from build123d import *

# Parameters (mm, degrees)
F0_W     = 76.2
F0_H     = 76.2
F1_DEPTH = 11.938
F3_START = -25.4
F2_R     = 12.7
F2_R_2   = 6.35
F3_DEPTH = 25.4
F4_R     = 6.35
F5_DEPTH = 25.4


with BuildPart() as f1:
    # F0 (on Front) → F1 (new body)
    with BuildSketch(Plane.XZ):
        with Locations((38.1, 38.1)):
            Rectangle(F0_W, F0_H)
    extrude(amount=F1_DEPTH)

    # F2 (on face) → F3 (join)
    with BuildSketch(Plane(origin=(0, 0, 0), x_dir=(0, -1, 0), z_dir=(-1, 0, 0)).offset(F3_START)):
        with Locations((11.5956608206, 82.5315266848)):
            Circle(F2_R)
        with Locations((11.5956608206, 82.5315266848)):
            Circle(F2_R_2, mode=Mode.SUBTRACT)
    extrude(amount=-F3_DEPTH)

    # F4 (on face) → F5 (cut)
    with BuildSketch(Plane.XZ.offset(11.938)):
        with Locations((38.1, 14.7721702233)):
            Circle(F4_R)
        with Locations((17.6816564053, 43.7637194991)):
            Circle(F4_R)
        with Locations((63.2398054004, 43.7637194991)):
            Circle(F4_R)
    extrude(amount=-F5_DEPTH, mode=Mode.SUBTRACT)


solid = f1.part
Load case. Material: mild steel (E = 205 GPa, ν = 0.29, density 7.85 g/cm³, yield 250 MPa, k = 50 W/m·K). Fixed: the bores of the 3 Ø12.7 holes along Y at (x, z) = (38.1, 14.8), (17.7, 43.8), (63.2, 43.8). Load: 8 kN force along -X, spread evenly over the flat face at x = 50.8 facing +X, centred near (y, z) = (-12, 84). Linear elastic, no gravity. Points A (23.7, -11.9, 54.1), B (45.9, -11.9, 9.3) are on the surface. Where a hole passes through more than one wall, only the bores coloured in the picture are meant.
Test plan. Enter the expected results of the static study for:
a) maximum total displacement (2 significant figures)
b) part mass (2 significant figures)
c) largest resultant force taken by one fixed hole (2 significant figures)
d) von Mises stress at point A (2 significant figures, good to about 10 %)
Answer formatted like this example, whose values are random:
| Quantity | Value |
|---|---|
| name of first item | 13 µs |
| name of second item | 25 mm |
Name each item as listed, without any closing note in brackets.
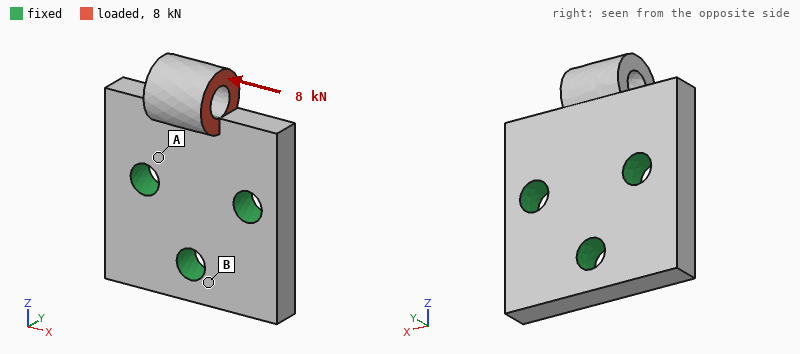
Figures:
| Quantity | Value |
|---|---|
| maximum total displacement | 27 µm |
| part mass | 570 g |
| largest resultant force taken by one fixed hole | 7.2 kN |
| von Mises stress at point A | 30 MPa |
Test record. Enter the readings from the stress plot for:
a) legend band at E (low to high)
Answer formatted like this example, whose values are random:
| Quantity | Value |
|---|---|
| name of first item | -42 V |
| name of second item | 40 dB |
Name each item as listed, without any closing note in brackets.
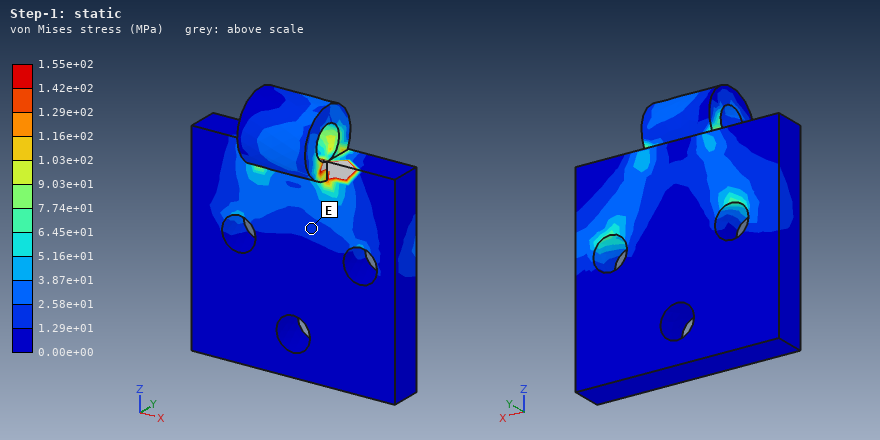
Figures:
| Quantity | Value |
|---|---|
| legend band at E | 1.29e+01 to 2.58e+01 MPa |
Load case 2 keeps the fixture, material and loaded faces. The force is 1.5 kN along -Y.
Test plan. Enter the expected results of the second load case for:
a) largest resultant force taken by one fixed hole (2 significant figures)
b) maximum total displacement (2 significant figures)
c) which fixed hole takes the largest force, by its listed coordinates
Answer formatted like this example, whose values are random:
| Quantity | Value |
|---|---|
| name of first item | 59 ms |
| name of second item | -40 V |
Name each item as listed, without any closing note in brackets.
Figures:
| Quantity | Value |
|---|---|
| largest resultant force taken by one fixed hole | 1.2 kN |
| maximum total displacement | 31 µm |
| which fixed hole takes the largest force, by its listed coordinates | (63.2, 43.8) |
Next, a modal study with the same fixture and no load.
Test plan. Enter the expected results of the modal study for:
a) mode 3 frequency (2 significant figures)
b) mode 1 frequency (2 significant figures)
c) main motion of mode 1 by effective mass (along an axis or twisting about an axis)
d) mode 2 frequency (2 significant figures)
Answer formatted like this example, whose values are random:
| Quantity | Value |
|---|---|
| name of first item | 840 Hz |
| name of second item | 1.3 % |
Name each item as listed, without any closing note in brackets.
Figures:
| Quantity | Value |
|---|---|
| mode 3 frequency | 11 kHz |
| mode 1 frequency | 4600 Hz |
| main motion of mode 1 by effective mass | along Y |
| mode 2 frequency | 11 kHz |
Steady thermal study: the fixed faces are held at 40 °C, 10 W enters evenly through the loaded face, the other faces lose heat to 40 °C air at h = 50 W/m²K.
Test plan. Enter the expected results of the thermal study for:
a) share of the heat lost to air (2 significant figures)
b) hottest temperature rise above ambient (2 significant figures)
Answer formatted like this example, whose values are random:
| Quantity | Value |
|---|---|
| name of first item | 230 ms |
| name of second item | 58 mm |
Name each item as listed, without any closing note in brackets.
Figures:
| Quantity | Value |
|---|---|
| share of the heat lost to air | 25 % |
| hottest temperature rise above ambient | 19 K |
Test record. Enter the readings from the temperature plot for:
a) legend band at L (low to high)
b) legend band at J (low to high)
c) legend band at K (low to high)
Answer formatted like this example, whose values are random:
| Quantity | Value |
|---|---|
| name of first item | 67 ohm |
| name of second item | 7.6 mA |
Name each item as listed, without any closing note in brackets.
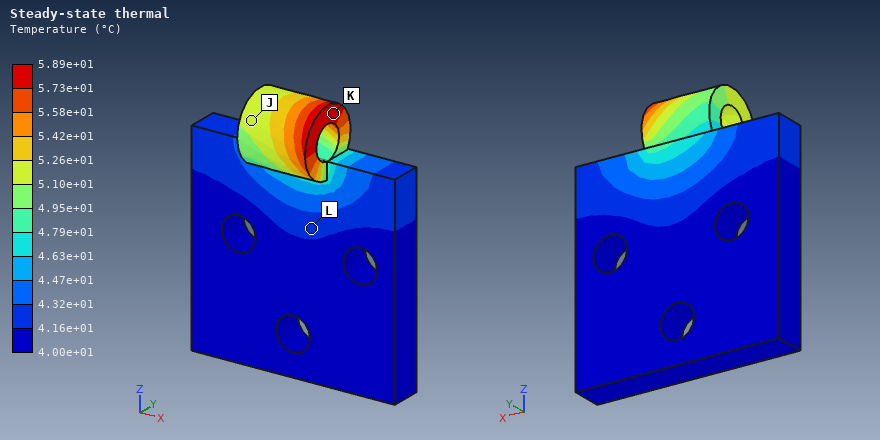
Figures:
| Quantity | Value |
|---|---|
| legend band at L | 4.16e+01 to 4.32e+01 °C |
| legend band at J | 5.10e+01 to 5.26e+01 °C |
| legend band at K | 5.73e+01 to 5.89e+01 °C |
